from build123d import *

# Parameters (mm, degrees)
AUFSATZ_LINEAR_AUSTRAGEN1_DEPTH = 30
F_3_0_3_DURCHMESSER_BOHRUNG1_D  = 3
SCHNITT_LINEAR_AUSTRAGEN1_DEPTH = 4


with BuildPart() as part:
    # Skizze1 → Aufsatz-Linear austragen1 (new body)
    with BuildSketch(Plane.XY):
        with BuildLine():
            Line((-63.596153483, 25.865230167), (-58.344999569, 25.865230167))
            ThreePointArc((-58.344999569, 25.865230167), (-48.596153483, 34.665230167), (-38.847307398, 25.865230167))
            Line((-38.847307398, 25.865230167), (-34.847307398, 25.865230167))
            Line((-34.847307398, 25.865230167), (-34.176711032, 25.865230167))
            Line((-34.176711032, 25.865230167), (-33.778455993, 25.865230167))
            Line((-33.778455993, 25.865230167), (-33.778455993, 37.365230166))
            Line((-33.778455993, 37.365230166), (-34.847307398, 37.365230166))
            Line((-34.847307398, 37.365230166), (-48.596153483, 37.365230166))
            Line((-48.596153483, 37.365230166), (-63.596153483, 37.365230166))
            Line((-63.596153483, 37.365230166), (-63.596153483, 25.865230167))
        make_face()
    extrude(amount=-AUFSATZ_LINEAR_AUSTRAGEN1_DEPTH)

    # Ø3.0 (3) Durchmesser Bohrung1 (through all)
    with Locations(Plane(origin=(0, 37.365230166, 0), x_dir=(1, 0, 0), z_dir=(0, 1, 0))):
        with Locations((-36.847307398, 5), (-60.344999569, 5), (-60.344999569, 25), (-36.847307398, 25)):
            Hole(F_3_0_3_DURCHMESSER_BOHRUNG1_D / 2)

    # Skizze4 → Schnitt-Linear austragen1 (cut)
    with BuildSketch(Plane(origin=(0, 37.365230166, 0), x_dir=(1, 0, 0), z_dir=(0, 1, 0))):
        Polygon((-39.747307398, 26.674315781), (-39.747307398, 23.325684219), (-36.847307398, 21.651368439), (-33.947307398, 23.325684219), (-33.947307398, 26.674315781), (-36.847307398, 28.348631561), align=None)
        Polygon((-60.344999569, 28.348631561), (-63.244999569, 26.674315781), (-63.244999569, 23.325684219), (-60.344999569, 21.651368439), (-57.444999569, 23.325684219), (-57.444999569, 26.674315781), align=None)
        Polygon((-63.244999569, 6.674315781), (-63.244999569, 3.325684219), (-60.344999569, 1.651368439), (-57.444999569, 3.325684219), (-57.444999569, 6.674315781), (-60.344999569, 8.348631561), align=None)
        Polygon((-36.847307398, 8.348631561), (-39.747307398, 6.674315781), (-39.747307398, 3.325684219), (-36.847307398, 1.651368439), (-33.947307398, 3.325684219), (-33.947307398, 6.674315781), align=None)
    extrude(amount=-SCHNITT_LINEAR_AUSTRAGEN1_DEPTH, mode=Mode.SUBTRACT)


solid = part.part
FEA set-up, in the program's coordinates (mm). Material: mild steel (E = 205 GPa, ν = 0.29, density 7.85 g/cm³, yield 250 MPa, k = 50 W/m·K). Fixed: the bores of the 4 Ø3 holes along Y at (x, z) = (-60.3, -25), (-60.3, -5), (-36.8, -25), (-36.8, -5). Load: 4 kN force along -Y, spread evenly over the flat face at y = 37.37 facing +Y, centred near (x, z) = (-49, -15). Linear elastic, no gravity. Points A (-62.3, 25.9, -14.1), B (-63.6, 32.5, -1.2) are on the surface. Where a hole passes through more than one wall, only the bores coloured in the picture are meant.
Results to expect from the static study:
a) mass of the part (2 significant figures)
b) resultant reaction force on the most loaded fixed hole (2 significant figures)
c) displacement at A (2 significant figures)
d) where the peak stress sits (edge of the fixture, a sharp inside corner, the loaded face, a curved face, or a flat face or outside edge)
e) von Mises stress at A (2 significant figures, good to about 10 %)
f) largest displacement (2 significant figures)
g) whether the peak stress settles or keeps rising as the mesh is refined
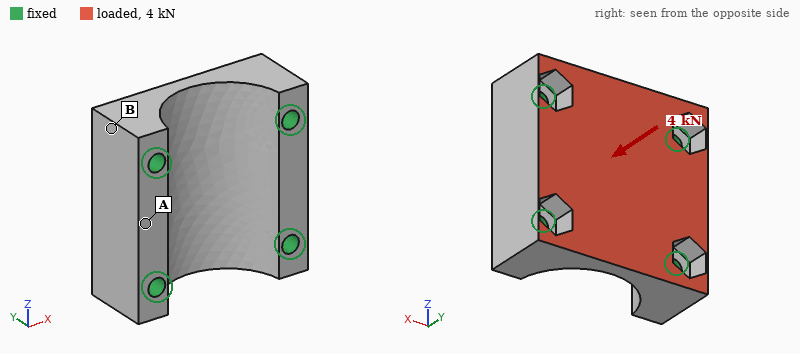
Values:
45 g
1.2 kN
0.99 µm
edge of the fixture
13 MPa
3.0 µm
keeps rising
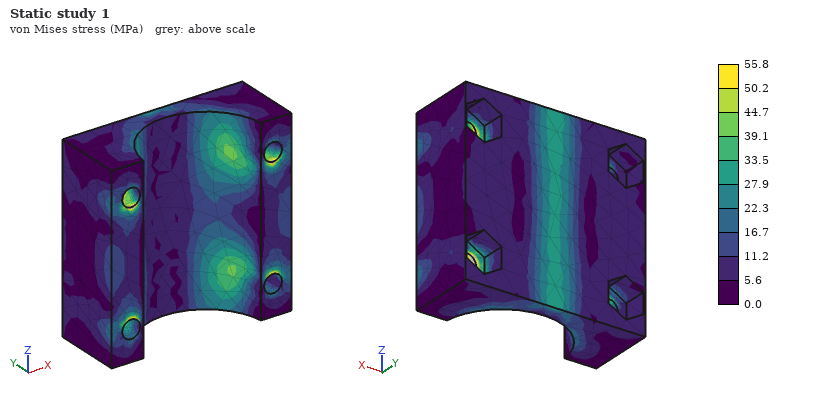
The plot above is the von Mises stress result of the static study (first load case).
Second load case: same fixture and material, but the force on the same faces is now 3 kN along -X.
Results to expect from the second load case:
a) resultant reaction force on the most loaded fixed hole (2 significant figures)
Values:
820 N
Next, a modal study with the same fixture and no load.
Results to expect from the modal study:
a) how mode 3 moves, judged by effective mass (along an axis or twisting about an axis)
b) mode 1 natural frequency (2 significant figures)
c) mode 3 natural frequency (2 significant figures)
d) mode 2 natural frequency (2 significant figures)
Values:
along Z
44 kHz
52 kHz
45 kHz
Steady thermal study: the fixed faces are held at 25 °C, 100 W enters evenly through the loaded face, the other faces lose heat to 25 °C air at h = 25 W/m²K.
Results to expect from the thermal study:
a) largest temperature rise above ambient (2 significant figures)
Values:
65 K
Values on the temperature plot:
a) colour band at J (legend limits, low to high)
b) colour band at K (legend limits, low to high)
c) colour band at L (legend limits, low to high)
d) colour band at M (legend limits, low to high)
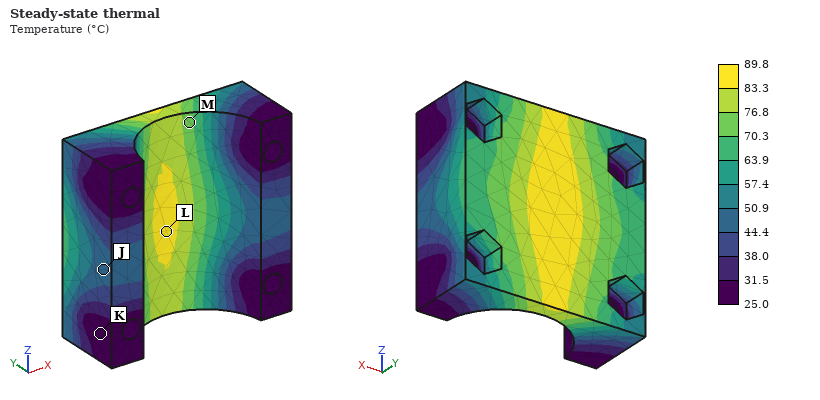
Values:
44.4 to 50.9 °C
25.0 to 31.5 °C
83.3 to 89.8 °C
70.3 to 76.8 °C
